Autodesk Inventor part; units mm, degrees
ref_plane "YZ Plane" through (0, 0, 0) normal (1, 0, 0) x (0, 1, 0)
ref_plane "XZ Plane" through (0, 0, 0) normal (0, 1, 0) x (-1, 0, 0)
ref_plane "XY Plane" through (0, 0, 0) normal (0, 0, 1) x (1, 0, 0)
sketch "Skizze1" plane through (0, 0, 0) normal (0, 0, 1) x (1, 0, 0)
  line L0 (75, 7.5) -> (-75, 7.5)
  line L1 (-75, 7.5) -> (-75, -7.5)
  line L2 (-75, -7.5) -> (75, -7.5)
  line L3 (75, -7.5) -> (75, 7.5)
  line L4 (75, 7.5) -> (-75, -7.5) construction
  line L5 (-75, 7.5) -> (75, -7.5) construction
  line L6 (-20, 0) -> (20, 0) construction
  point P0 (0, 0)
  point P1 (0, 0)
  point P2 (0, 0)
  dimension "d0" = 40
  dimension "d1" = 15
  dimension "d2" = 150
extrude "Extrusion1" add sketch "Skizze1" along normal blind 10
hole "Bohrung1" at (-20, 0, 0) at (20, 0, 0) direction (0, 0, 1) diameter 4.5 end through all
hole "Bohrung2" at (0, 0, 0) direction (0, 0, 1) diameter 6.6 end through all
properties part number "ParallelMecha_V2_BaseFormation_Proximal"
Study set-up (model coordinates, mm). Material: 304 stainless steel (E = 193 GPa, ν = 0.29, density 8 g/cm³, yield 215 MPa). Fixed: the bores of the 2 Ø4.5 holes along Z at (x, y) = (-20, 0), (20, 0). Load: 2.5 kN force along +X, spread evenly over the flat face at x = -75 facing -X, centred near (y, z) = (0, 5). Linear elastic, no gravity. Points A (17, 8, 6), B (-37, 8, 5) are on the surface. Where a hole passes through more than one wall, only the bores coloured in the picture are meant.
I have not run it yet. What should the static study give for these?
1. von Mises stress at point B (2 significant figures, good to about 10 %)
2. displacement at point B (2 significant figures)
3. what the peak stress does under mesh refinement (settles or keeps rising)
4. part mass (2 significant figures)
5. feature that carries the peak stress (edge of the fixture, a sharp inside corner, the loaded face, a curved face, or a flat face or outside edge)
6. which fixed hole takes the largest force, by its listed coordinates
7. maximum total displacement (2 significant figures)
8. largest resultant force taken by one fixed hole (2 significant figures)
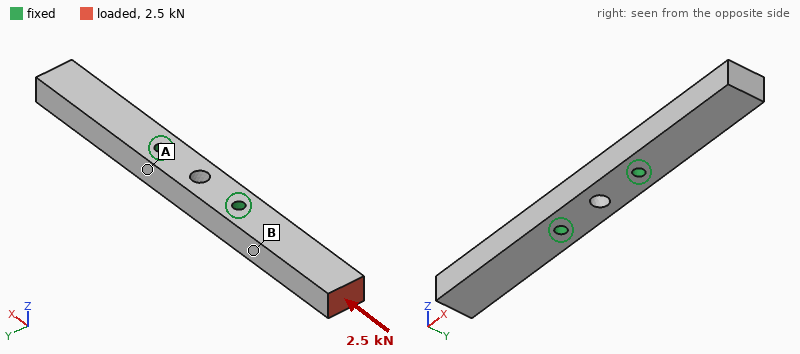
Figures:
17 MPa
1.5 µm
keeps rising
170 g
edge of the fixture
(-20, 0)
4.8 µm
2.4 kN
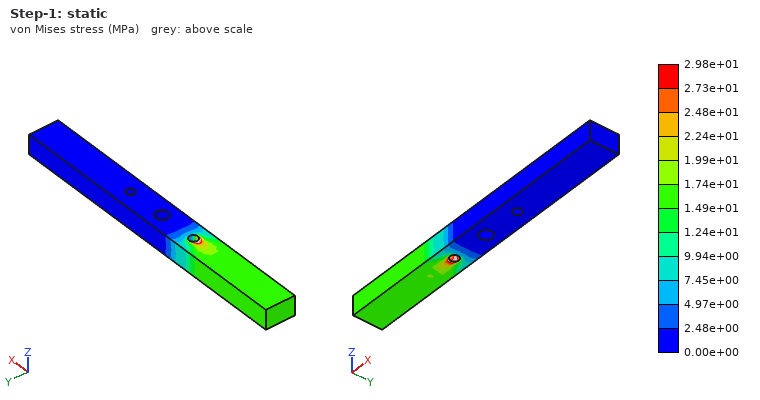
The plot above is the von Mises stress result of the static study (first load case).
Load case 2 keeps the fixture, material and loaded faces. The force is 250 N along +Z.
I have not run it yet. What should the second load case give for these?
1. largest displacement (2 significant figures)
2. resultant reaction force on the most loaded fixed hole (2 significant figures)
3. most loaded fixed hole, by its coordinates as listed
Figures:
59 µm
290 N
(-20, 0)
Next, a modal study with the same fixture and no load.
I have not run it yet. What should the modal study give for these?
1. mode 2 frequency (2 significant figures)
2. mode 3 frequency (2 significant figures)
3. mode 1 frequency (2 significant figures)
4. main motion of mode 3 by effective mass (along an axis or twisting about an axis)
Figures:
2600 Hz
3100 Hz
2600 Hz
along Y
